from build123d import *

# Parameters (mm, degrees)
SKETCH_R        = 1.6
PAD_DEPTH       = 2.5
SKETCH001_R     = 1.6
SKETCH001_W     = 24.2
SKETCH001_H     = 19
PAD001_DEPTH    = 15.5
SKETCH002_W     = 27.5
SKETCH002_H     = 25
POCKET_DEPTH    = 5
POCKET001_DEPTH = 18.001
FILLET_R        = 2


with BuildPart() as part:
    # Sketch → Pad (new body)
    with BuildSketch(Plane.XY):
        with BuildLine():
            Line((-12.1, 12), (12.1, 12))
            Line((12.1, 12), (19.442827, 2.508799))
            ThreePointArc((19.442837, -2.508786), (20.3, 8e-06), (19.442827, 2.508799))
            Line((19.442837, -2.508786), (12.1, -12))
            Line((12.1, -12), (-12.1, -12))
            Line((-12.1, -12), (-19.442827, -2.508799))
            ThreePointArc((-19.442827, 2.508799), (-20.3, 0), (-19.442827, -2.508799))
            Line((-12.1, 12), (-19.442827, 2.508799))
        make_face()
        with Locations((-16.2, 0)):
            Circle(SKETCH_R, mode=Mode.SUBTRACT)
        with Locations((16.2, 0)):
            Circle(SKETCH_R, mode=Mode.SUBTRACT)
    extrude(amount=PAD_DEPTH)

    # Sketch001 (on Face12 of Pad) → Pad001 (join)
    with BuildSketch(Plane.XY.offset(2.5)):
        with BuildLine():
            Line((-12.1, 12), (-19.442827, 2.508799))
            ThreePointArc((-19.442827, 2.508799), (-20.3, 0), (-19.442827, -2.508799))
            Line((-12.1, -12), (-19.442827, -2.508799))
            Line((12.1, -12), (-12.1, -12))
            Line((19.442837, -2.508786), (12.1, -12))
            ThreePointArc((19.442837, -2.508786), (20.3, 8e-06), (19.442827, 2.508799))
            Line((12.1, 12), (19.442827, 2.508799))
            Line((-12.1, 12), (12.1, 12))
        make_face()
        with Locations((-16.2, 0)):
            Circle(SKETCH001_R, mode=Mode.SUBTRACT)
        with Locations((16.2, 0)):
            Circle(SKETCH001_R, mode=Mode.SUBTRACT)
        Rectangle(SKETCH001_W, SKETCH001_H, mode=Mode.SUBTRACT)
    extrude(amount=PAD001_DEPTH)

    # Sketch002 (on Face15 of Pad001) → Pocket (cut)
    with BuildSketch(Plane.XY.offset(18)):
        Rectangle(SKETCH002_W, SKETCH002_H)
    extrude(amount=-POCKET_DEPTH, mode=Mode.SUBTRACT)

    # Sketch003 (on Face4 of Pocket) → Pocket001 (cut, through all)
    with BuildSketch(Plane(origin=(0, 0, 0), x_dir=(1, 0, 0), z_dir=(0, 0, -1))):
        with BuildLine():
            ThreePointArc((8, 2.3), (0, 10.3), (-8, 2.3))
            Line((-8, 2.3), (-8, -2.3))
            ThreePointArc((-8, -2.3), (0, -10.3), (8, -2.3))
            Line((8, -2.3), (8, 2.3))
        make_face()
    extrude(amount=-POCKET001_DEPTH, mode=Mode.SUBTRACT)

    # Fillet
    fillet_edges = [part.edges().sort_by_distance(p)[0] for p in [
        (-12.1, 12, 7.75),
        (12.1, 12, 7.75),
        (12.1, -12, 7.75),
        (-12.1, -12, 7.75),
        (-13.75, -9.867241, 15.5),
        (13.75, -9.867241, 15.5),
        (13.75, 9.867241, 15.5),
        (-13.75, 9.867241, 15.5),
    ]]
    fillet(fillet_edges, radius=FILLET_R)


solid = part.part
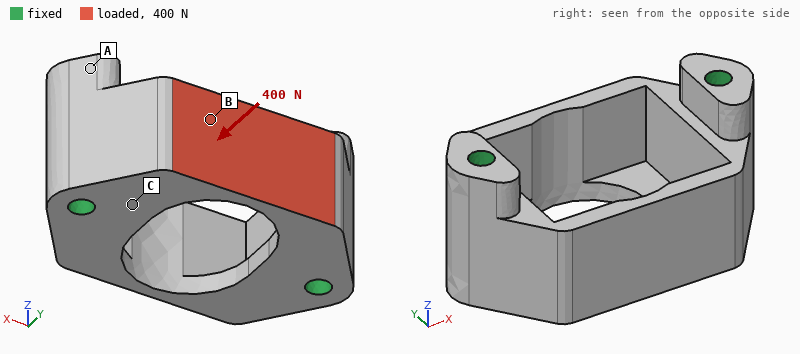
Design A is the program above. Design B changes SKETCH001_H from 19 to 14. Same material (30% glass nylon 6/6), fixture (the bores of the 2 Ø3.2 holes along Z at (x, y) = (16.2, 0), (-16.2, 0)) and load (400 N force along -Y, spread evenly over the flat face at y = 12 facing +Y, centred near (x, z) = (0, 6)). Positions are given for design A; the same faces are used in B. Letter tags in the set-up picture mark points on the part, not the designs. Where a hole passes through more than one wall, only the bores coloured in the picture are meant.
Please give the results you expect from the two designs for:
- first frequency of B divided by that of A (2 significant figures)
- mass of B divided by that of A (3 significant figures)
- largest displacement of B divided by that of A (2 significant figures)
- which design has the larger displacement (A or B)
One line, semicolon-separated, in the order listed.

1.3; 1.14; 0.27; A
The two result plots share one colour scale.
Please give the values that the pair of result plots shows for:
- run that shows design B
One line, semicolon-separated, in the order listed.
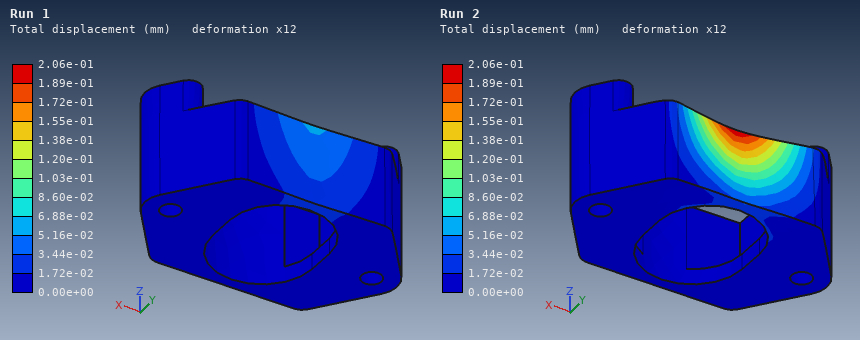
Run 1
